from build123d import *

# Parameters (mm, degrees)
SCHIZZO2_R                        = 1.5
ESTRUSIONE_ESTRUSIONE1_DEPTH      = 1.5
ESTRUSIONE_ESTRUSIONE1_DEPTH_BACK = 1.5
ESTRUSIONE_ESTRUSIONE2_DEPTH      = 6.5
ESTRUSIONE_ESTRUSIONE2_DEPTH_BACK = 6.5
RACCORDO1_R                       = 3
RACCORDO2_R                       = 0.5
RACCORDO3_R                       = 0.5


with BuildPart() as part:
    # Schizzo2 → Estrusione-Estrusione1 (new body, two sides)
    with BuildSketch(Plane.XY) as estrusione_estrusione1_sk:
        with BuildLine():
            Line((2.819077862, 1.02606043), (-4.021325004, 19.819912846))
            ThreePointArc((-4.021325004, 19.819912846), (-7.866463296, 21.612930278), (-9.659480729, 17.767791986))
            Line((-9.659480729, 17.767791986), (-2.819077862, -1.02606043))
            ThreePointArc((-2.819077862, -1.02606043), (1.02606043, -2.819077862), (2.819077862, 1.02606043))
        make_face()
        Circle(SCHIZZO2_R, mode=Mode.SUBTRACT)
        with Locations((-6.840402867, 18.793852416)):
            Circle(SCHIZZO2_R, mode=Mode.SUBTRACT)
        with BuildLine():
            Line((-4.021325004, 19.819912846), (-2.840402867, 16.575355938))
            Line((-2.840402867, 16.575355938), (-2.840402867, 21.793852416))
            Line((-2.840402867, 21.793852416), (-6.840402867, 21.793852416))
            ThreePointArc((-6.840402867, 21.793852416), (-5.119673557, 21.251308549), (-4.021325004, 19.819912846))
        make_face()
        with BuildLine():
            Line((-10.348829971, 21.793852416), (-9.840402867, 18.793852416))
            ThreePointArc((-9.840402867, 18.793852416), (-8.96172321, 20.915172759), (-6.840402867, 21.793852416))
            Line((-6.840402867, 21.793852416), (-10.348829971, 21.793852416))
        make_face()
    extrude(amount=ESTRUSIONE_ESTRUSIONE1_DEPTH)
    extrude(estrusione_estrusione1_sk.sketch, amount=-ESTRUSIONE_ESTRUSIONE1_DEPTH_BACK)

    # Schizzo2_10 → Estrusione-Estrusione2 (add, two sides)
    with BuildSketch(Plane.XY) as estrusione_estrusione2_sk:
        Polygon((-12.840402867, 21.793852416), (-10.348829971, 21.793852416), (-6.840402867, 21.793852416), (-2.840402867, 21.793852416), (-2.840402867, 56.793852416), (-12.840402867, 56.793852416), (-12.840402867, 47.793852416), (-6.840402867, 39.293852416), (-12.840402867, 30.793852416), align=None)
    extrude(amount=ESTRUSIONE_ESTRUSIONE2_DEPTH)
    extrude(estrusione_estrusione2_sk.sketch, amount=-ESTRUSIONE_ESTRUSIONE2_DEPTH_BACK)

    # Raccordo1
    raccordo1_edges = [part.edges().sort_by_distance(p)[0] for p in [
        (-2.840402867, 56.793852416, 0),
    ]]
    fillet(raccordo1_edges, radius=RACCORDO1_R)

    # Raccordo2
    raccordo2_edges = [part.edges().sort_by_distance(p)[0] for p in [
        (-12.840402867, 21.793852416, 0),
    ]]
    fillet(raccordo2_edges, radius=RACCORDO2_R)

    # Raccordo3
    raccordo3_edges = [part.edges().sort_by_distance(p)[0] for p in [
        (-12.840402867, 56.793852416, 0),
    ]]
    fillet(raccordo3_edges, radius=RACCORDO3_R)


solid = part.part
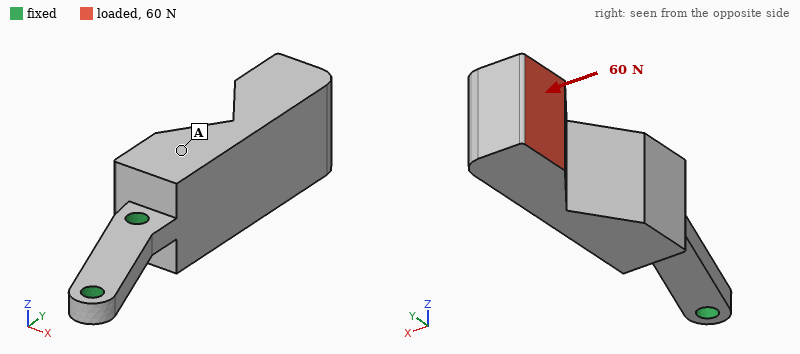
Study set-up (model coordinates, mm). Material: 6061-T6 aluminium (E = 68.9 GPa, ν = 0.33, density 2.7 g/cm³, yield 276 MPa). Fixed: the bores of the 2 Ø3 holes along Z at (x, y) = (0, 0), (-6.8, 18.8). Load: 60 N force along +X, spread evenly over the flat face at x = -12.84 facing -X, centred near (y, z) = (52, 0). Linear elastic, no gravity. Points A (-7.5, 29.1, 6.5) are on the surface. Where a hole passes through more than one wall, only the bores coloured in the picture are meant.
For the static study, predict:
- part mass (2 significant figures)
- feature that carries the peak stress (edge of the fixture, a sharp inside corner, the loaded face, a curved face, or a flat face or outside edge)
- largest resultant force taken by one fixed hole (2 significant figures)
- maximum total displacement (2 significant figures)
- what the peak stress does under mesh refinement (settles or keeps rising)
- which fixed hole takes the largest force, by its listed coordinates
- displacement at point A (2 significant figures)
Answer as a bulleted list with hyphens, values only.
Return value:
- 12 g
- edge of the fixture
- 79 N
- 86 µm
- keeps rising
- (-6.8, 18.8)
- 15 µm
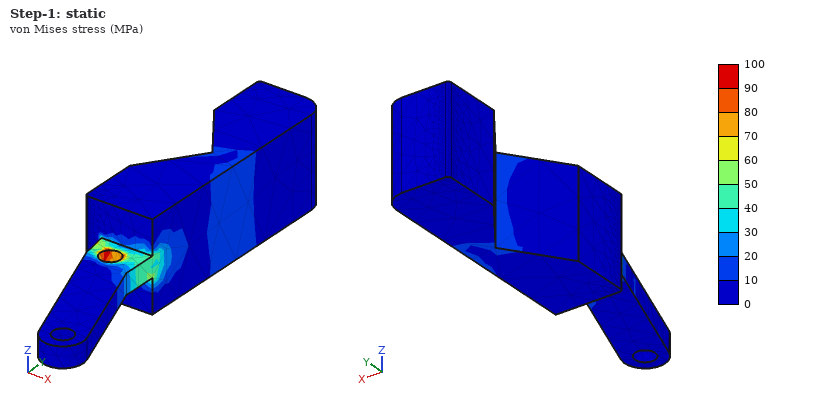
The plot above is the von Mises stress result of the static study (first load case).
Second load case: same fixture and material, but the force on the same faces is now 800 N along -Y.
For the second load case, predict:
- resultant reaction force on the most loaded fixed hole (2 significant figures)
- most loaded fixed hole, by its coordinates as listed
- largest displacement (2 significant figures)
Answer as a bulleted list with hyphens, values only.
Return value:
- 850 N
- (-6.8, 18.8)
- 0.31 mm
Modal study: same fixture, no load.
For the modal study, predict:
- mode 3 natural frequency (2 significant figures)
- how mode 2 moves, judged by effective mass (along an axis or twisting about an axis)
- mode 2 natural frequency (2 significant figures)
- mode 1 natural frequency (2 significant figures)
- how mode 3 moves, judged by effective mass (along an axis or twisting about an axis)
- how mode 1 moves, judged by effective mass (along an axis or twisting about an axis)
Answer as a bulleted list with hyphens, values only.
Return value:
- 7600 Hz
- along X
- 2100 Hz
- 1400 Hz
- twisting about Y
- along Z
